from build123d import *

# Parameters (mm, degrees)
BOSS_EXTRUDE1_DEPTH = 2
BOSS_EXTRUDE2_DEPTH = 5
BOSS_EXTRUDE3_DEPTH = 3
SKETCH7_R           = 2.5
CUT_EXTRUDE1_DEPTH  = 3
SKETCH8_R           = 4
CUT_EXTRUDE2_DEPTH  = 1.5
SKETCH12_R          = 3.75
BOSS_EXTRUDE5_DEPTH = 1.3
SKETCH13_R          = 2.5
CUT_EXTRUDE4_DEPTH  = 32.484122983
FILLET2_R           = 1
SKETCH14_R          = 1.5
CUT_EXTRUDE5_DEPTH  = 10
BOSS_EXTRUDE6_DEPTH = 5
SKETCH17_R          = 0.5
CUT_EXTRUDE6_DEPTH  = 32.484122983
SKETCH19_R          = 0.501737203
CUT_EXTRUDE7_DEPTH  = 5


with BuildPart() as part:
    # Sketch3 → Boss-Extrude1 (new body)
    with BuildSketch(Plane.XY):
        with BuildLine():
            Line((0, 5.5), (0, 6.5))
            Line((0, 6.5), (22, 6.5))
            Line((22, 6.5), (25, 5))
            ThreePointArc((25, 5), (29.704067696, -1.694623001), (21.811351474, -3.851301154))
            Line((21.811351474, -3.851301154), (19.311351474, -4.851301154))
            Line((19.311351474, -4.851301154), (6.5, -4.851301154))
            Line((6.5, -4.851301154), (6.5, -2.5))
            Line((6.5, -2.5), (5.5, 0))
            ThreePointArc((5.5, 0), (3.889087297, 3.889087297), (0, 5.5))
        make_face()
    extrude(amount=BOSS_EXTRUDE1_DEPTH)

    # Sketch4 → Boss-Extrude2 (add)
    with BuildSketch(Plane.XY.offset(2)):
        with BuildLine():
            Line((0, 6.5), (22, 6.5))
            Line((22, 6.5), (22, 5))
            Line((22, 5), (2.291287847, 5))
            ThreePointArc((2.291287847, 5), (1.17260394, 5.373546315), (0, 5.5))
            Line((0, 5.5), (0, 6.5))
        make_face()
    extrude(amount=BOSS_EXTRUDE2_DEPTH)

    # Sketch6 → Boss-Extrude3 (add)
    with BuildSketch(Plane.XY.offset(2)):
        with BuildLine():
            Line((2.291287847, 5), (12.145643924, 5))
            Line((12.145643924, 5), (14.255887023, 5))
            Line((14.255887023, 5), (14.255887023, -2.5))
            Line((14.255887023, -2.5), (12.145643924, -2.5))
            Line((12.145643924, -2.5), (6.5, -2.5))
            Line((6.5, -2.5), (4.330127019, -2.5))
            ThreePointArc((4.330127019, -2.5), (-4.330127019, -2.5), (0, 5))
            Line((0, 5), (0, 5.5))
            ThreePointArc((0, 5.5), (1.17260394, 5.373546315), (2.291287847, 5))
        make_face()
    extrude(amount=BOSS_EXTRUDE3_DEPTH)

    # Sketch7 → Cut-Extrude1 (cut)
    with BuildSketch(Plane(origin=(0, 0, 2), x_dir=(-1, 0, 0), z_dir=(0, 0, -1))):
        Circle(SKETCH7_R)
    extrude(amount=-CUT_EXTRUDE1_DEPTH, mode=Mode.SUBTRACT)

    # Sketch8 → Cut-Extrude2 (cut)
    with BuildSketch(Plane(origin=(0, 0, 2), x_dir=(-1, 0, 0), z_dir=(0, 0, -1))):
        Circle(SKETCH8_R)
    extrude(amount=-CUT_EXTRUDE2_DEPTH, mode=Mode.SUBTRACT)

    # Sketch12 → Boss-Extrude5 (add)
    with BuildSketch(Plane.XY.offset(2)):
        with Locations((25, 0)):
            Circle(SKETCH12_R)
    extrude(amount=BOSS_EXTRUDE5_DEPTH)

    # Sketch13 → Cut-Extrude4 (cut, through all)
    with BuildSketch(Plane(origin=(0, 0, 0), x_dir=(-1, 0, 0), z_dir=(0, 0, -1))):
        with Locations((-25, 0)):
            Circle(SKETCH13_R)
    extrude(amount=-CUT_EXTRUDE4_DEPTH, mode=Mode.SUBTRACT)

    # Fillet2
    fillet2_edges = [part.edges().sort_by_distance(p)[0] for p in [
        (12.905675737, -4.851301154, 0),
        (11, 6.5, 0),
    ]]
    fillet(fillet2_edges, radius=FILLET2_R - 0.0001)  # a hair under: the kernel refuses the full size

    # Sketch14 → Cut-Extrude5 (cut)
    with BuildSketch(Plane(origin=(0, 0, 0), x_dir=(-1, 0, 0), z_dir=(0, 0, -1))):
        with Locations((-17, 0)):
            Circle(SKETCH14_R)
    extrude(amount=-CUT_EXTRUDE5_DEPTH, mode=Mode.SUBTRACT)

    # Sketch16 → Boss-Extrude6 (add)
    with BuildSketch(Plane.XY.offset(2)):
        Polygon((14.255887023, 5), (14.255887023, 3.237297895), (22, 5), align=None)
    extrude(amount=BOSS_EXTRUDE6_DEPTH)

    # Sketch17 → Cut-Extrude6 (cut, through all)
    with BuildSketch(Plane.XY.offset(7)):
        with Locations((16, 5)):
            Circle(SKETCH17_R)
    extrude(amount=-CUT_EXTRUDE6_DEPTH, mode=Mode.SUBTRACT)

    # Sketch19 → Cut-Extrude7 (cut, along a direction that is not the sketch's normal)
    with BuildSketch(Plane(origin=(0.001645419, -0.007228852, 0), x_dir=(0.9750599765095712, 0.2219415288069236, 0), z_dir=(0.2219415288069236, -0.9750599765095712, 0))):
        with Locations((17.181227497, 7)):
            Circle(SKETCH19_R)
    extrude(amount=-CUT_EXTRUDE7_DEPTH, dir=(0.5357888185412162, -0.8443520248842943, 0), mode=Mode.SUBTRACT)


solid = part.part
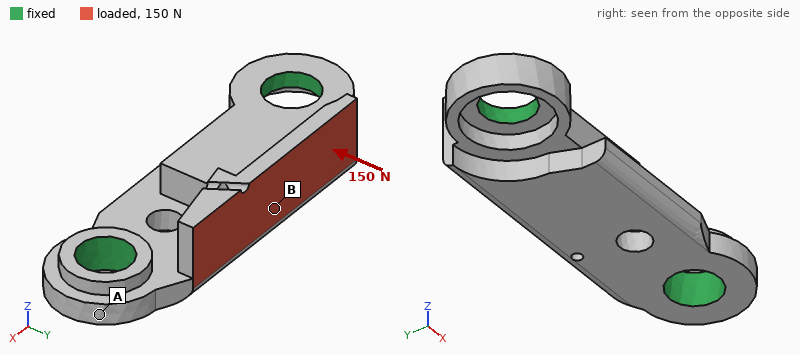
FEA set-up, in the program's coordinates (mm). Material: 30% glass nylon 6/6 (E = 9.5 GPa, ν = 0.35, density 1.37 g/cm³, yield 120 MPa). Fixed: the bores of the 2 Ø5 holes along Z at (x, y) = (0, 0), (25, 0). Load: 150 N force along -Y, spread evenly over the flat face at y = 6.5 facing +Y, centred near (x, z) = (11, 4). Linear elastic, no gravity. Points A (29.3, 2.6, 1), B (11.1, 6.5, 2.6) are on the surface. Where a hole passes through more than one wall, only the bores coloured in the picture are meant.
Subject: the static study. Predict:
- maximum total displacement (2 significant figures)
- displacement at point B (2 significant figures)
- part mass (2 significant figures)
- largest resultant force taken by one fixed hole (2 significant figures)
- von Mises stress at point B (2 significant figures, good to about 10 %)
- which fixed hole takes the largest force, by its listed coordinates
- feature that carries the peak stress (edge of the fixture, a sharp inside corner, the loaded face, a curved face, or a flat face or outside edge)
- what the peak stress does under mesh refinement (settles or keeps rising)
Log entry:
50 µm
22 µm
1.4 g
93 N
6.1 MPa
(0, 0)
edge of the fixture
keeps rising
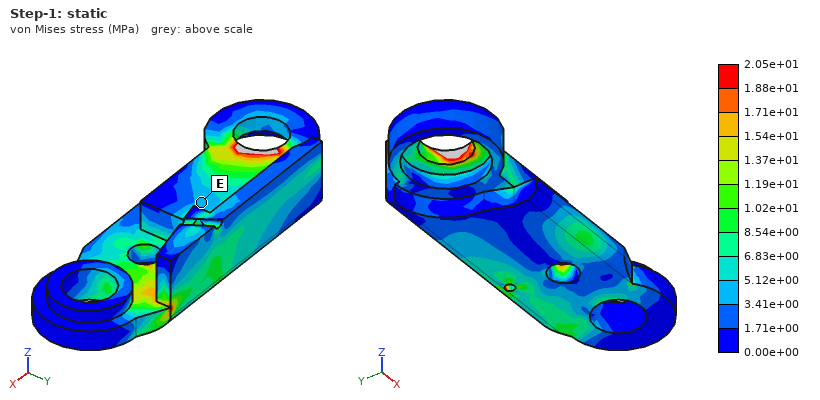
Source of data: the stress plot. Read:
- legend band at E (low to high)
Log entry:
3.41e+00 to 5.12e+00 MPa
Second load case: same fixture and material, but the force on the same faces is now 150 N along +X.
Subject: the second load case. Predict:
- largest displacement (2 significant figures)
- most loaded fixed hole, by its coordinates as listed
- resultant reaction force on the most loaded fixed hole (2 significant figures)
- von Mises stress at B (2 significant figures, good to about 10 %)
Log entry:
24 µm
(0, 0)
95 N
2.6 MPa
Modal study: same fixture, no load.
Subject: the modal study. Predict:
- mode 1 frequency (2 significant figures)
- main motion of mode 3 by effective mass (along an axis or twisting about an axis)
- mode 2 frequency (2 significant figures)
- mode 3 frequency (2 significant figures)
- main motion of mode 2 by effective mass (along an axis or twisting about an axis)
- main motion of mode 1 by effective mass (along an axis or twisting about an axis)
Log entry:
10 kHz
along Y
13 kHz
18 kHz
along Z
along Z
